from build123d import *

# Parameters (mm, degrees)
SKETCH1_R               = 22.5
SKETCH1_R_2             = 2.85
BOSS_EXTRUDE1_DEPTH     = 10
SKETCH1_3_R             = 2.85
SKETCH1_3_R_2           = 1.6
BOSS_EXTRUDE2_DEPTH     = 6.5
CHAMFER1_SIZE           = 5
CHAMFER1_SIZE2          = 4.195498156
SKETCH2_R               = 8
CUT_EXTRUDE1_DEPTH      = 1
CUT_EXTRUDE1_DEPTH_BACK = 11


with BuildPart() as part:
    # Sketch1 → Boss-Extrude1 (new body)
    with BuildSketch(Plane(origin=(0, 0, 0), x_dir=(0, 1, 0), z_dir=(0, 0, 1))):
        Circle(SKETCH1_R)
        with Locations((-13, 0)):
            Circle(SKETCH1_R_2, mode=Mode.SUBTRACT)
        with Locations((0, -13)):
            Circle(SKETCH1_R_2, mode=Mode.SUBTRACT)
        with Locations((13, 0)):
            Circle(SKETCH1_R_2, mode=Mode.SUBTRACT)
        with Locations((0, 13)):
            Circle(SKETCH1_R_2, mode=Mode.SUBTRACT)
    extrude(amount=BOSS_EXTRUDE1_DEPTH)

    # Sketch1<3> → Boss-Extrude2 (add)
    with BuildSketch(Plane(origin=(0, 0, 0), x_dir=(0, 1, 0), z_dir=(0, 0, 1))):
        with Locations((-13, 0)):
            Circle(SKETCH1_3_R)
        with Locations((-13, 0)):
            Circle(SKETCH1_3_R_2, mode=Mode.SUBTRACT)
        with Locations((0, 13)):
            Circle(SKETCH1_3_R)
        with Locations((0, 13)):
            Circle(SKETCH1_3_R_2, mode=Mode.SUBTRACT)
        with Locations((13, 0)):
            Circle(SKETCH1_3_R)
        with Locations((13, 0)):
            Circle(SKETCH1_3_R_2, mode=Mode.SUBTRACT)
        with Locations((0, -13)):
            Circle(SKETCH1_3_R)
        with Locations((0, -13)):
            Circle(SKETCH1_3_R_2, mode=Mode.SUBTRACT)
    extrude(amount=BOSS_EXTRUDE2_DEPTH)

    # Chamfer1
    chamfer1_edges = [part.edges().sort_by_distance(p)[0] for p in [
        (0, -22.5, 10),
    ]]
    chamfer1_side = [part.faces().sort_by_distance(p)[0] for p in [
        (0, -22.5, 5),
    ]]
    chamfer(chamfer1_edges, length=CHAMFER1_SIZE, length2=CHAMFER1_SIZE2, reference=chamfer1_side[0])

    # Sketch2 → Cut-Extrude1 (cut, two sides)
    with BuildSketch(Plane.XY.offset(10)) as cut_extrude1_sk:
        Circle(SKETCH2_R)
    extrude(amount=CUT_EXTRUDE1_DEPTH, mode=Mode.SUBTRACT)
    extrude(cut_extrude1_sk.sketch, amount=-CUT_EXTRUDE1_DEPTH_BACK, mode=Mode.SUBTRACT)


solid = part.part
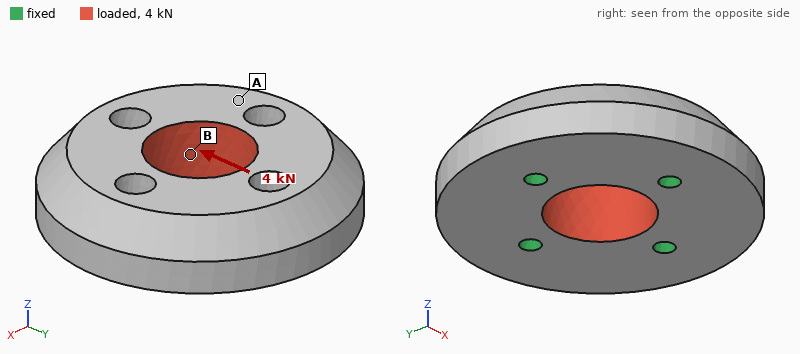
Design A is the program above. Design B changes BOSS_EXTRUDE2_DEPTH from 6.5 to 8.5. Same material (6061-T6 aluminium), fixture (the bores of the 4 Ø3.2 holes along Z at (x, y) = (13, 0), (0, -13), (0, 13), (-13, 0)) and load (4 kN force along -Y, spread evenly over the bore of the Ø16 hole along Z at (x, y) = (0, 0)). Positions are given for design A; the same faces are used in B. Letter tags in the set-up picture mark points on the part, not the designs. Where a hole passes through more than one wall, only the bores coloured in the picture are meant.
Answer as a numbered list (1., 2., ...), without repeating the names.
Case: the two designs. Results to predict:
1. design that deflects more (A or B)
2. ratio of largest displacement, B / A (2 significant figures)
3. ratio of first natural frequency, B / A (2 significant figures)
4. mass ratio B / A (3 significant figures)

1. A
2. 0.55
3. 1.2
4. 1.01
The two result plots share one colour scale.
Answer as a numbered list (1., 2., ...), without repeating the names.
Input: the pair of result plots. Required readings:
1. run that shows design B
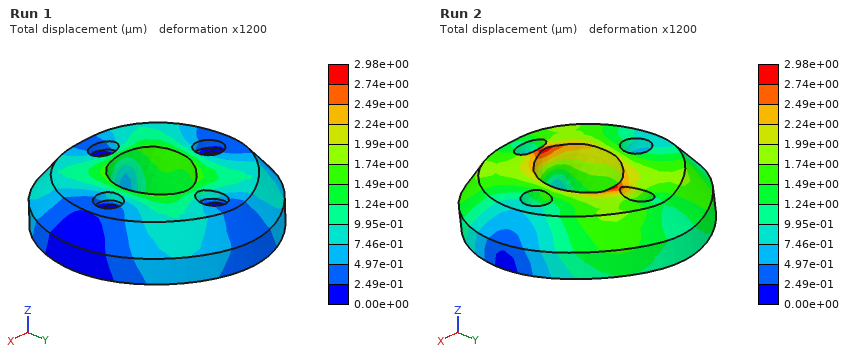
1. Run 1
